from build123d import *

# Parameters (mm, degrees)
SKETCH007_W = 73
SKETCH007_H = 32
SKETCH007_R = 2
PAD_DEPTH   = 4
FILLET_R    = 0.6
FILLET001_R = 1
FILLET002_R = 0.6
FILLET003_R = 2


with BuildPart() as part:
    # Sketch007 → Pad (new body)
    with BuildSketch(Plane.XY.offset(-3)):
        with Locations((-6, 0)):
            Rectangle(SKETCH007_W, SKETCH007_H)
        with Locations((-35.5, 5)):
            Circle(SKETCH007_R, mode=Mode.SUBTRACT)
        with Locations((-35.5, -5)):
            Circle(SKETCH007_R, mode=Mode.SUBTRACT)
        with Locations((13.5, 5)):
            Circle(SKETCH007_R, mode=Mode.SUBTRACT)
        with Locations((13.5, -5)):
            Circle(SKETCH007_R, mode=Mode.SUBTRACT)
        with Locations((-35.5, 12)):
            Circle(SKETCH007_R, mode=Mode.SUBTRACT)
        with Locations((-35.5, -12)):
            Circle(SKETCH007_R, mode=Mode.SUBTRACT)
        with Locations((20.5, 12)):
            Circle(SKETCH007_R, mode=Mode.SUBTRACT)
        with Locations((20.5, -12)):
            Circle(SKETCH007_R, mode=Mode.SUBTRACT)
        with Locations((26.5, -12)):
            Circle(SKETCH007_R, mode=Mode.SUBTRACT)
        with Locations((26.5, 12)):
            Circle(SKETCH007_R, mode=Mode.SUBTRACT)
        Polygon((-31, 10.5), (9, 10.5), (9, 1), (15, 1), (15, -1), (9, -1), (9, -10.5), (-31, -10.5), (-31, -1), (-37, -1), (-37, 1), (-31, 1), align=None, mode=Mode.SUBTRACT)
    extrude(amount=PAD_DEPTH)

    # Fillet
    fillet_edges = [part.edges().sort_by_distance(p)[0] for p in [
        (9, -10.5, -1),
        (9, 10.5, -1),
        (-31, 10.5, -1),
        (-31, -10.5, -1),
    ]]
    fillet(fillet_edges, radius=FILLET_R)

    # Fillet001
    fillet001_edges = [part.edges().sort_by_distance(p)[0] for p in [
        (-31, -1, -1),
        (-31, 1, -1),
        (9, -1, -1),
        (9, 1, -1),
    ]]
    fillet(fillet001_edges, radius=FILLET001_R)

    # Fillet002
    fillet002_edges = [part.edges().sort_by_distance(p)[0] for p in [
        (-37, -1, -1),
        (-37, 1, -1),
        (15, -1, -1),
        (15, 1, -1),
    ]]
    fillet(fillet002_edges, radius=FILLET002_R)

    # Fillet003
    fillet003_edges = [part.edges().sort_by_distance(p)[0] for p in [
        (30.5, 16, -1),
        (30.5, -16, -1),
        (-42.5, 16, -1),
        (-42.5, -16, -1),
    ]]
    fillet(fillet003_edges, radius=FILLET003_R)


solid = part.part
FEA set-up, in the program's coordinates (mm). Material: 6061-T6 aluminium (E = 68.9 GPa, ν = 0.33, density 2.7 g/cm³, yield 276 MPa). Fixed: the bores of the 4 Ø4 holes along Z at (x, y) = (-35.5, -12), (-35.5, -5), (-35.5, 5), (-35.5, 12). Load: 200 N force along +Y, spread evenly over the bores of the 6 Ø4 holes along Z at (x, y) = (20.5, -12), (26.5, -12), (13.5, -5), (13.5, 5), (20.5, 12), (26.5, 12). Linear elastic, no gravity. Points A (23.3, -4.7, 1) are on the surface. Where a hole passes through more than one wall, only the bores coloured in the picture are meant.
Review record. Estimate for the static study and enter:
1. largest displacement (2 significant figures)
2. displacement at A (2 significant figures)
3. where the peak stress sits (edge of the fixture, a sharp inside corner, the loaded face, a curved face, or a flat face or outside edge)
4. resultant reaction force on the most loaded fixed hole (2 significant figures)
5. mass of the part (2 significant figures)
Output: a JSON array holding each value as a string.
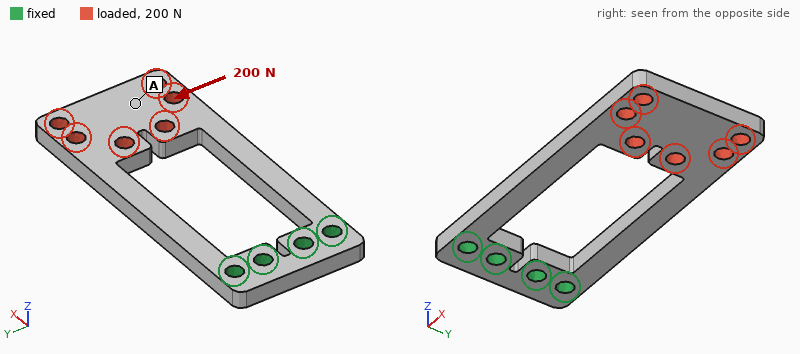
["0.24 mm", "0.24 mm", "a curved face", "390 N", "15 g"]
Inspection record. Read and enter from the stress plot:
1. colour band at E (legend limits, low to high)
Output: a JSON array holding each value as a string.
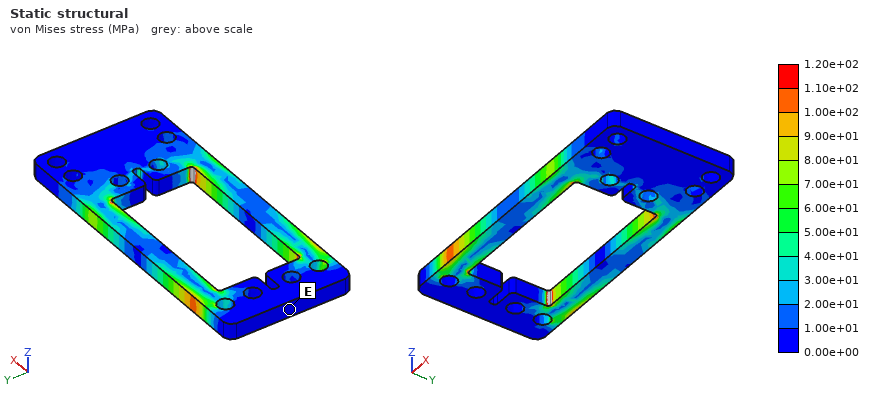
["0.00e+00 to 1.00e+01 MPa"]
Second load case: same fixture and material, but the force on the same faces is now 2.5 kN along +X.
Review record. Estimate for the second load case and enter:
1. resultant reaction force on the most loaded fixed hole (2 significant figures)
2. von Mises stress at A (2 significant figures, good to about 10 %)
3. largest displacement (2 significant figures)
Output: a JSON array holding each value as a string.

["1.3 kN", "15 MPa", "55 µm"]
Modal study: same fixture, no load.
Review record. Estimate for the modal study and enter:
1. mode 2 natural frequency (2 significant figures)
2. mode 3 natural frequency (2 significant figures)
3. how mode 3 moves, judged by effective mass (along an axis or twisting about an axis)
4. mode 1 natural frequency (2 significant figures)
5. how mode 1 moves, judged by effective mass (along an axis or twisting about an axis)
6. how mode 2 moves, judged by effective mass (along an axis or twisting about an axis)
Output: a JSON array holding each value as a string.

["1600 Hz", "2000 Hz", "twisting about X", "530 Hz", "along Z", "along Y"]
